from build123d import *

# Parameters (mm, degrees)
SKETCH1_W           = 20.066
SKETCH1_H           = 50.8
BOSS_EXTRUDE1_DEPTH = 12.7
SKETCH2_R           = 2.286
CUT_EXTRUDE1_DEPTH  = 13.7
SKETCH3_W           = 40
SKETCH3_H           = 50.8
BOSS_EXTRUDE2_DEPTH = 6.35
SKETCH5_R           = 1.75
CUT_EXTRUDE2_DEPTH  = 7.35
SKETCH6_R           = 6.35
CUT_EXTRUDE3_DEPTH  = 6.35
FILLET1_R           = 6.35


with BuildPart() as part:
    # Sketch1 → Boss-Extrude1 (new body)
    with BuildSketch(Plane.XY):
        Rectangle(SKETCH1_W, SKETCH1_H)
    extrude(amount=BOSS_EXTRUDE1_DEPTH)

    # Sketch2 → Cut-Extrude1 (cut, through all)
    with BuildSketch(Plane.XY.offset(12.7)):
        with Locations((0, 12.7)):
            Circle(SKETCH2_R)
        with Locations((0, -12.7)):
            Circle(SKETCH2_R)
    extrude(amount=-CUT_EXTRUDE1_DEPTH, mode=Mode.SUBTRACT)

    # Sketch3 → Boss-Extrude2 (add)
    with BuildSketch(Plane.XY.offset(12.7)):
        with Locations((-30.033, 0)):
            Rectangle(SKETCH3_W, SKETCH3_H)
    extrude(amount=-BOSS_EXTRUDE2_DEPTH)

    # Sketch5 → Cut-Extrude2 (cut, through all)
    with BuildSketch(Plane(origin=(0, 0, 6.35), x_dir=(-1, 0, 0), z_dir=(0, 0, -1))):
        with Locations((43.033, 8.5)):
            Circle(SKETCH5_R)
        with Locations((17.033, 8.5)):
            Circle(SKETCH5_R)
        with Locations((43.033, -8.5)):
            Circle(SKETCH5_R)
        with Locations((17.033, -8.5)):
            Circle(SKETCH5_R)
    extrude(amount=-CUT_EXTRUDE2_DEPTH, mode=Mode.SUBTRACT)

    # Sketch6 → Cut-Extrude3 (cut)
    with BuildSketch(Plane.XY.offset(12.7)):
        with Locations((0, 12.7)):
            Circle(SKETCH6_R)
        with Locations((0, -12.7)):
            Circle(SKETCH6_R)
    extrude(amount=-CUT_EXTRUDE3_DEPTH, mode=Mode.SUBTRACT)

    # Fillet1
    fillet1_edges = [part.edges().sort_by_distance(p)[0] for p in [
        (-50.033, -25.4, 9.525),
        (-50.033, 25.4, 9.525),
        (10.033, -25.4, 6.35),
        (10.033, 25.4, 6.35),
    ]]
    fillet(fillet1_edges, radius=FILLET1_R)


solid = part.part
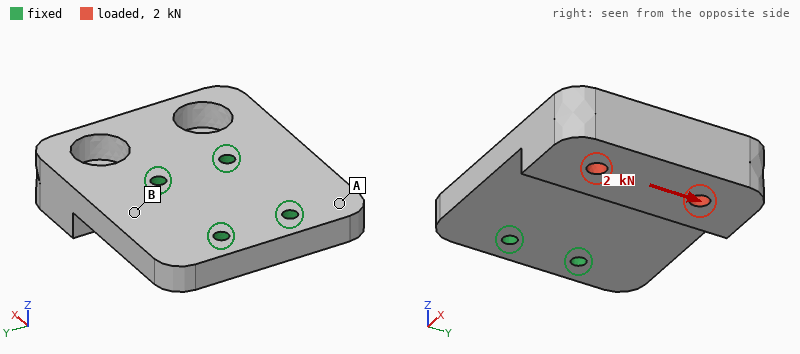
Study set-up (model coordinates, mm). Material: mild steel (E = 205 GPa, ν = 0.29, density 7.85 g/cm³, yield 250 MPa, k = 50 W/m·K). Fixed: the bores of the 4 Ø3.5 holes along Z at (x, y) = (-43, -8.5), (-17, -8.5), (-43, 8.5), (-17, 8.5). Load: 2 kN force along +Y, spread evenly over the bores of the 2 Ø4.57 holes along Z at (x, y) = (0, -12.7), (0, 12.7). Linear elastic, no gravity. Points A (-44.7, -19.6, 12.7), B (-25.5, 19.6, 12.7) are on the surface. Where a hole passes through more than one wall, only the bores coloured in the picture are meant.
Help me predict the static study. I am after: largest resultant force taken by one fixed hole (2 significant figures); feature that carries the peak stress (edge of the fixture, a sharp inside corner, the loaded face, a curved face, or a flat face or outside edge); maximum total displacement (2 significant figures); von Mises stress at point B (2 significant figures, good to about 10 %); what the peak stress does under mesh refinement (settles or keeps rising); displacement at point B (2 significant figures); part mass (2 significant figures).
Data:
1.6 kN
edge of the fixture
6.0 µm
12 MPa
keeps rising
1.2 µm
180 g
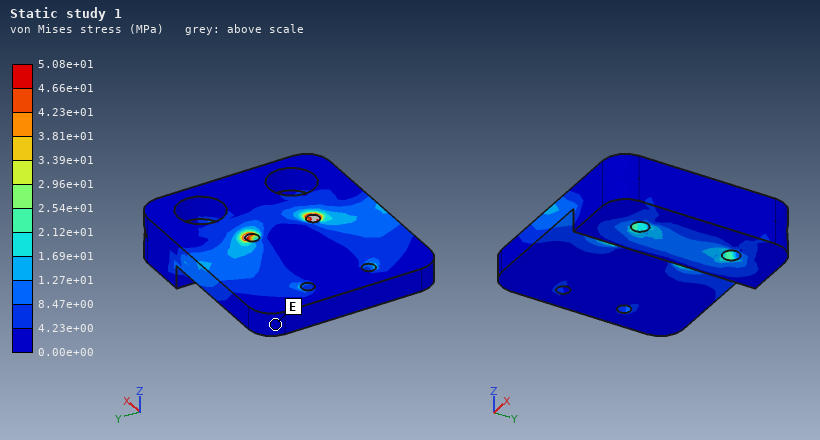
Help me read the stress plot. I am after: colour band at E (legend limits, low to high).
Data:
0.00e+00 to 4.23e+00 MPa
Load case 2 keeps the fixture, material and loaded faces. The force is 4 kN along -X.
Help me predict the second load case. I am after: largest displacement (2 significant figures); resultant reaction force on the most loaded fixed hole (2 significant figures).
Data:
34 µm
1.7 kN
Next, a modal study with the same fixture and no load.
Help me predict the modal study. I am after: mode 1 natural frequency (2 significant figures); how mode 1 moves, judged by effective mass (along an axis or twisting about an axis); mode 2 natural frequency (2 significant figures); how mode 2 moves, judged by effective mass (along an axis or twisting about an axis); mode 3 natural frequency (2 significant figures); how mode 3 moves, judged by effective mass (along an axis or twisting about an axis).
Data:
4800 Hz
along Z
8100 Hz
twisting about X
13 kHz
along Y
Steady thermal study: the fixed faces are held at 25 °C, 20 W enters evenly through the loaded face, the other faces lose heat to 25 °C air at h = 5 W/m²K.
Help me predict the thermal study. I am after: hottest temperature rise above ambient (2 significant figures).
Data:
29 K
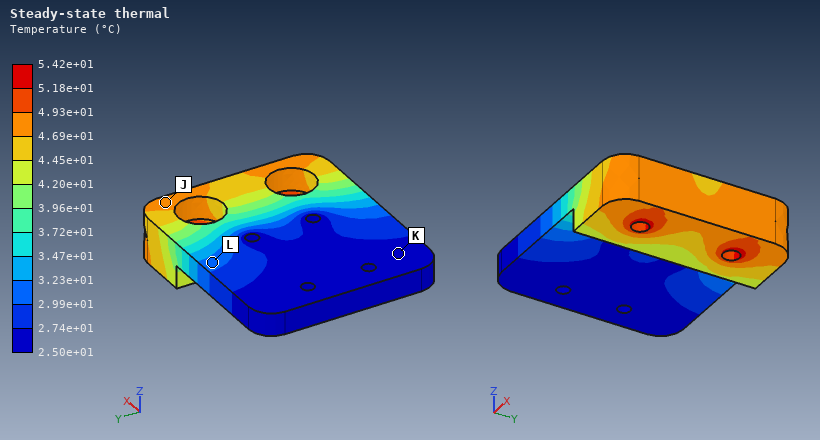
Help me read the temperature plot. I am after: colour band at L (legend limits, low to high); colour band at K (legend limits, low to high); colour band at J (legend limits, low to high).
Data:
2.99e+01 to 3.23e+01 °C
2.50e+01 to 2.74e+01 °C
4.69e+01 to 4.93e+01 °C
